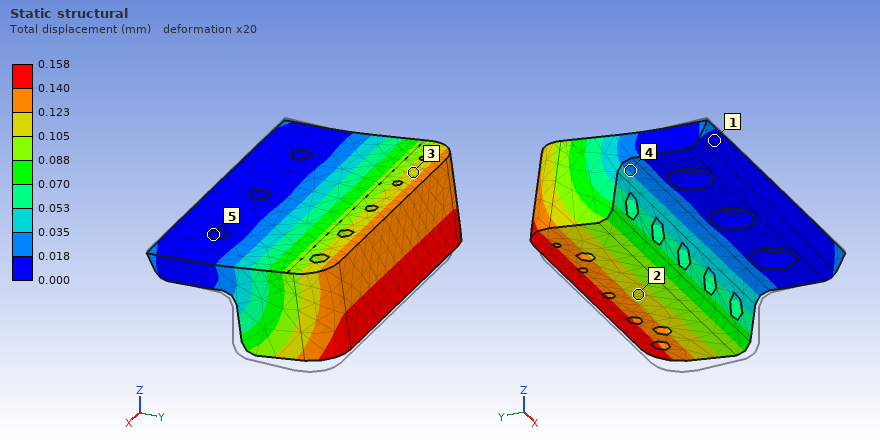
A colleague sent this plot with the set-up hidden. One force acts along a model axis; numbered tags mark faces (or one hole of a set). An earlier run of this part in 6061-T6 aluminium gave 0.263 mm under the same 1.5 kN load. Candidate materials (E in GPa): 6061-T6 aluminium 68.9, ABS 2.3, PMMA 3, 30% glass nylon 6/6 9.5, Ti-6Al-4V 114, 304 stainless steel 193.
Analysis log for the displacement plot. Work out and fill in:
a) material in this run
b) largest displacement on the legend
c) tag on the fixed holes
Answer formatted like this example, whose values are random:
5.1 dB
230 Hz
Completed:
Ti-6Al-4V
0.158 mm
5
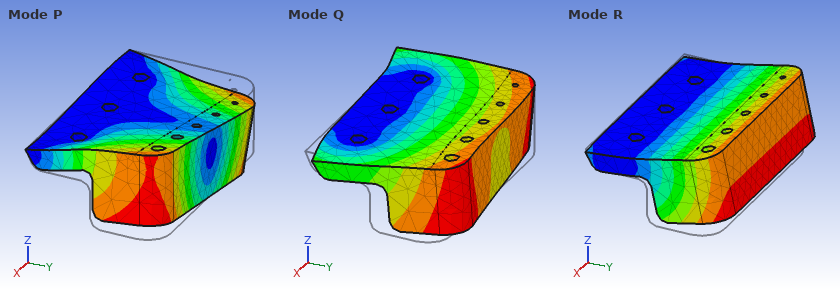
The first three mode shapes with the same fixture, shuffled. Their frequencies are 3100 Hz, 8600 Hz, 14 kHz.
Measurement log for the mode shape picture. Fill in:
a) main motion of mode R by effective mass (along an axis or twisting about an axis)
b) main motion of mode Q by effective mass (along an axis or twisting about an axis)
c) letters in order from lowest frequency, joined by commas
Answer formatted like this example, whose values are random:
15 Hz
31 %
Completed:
along Z
along X
R, P, Q
